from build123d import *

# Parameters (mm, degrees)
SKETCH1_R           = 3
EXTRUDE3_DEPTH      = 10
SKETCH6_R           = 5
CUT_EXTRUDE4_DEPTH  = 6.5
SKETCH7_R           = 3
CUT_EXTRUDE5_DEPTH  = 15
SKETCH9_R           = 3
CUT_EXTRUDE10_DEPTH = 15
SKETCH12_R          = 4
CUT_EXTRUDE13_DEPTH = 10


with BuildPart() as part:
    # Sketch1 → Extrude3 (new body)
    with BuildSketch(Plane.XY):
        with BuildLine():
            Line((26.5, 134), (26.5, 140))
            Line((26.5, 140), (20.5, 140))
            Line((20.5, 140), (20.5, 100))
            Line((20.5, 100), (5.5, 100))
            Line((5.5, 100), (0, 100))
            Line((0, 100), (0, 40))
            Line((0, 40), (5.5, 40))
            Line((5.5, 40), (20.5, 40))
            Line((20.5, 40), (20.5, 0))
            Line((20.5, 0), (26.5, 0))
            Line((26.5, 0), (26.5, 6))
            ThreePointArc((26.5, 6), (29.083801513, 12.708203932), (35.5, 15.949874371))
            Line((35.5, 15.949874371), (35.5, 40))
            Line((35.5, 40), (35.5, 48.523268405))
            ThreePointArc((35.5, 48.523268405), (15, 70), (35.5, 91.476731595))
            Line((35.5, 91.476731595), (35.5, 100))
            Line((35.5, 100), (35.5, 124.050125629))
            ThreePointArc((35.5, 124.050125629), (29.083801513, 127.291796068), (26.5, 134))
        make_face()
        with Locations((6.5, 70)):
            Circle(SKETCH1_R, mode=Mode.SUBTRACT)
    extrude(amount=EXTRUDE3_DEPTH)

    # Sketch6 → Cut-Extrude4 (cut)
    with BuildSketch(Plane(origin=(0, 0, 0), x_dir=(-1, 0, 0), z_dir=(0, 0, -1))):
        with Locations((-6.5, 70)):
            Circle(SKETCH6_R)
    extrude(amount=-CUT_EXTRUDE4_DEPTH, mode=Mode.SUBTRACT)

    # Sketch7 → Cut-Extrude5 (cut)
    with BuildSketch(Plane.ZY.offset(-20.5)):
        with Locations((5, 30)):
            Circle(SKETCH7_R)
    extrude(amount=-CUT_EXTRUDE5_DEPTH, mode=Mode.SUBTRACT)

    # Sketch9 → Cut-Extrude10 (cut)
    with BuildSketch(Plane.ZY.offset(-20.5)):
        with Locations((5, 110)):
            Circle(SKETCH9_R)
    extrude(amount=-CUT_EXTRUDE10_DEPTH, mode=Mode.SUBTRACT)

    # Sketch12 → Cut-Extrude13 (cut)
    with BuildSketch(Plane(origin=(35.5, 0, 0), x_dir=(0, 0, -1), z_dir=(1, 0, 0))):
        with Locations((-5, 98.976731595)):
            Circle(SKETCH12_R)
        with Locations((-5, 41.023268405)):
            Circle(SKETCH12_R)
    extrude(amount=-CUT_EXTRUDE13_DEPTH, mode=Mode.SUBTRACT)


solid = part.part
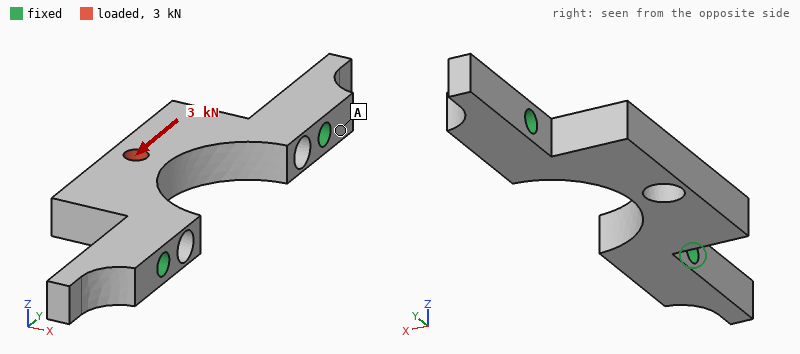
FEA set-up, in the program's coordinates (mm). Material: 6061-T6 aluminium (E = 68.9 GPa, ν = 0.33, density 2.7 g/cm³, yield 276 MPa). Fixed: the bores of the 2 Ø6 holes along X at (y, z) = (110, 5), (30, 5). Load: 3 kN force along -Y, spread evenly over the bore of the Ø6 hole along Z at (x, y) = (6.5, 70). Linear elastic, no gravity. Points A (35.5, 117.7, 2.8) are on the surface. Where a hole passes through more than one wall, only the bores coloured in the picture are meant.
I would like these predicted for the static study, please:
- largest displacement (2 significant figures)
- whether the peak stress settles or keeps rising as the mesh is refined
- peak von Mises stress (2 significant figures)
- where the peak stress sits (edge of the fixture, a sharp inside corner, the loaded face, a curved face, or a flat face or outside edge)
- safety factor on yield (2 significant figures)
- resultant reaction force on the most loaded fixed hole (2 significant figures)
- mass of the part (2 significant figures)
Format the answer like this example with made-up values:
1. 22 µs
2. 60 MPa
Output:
1. 21 µm
2. settles
3. 100 MPa
4. the loaded face
5. 2.8
6. 1.7 kN
7. 58 g
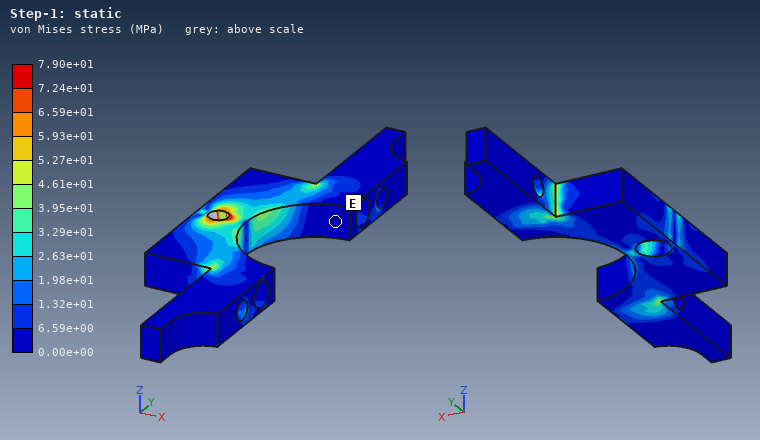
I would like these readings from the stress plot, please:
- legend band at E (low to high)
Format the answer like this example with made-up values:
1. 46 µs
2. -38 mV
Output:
1. 0.00e+00 to 6.59e+00 MPa
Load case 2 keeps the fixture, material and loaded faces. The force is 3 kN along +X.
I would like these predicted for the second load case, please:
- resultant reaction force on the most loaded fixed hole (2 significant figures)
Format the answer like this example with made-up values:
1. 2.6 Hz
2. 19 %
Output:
1. 2.3 kN
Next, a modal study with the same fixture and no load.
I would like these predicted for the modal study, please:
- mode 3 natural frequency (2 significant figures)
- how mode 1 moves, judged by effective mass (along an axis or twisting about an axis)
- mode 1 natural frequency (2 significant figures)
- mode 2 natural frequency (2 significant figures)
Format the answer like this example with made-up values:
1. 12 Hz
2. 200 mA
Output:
1. 11 kHz
2. along Z
3. 3800 Hz
4. 8600 Hz
